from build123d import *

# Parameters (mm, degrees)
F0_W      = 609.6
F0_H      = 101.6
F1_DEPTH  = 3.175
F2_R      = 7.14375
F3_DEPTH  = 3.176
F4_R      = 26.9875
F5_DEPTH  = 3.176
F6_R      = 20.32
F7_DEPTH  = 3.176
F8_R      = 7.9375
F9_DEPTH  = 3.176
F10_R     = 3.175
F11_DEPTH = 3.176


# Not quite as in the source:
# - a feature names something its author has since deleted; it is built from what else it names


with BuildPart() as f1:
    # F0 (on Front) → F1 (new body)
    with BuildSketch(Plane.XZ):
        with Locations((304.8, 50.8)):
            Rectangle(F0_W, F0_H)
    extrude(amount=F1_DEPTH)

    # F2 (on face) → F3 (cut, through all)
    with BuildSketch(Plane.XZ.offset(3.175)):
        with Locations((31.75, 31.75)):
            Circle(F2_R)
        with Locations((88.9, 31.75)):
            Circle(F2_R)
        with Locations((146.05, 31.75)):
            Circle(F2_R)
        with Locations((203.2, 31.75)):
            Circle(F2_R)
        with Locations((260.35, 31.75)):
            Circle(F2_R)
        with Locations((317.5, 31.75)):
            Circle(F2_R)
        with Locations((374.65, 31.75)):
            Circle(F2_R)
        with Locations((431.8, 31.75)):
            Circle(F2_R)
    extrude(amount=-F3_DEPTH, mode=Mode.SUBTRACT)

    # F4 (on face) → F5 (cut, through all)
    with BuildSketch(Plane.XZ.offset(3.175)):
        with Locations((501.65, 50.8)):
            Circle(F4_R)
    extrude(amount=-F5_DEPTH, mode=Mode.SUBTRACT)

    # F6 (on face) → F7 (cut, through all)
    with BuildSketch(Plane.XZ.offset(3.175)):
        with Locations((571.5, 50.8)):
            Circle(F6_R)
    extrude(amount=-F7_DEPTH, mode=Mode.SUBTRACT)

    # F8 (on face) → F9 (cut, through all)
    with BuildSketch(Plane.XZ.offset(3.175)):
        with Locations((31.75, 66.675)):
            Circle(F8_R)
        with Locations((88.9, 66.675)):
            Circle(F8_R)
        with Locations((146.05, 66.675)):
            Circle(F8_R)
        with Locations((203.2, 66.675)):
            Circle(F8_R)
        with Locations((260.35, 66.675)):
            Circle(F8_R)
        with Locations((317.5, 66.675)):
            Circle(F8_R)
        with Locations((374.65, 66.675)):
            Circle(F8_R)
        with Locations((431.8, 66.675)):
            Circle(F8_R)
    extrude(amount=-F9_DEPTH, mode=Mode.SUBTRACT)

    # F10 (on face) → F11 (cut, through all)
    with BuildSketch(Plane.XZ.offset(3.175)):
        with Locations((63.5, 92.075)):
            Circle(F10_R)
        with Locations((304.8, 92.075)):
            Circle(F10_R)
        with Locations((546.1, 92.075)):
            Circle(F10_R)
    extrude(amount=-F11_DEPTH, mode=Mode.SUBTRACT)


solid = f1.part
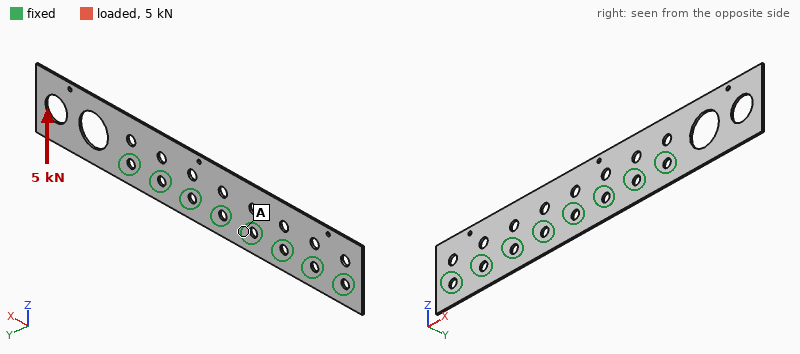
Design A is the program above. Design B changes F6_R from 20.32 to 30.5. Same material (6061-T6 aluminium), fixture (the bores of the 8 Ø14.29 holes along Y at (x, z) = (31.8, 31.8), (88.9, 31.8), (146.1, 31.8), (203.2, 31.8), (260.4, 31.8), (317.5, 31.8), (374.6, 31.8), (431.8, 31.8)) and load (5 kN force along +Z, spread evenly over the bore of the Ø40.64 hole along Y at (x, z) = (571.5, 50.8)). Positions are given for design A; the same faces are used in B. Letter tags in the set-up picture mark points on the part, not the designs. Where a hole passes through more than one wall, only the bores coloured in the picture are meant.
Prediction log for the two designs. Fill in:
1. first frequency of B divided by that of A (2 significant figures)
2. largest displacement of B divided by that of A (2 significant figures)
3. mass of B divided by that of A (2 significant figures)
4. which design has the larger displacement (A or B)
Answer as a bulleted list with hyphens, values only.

- 1.1
- 1.3
- 0.97
- B
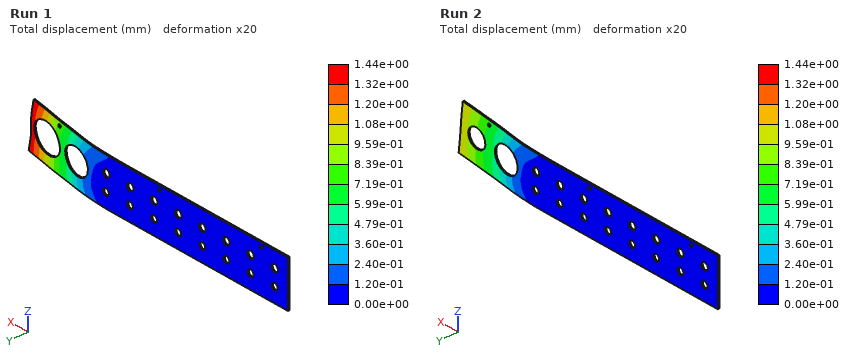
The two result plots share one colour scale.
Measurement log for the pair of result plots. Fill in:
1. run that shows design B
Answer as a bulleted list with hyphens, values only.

- Run 1
